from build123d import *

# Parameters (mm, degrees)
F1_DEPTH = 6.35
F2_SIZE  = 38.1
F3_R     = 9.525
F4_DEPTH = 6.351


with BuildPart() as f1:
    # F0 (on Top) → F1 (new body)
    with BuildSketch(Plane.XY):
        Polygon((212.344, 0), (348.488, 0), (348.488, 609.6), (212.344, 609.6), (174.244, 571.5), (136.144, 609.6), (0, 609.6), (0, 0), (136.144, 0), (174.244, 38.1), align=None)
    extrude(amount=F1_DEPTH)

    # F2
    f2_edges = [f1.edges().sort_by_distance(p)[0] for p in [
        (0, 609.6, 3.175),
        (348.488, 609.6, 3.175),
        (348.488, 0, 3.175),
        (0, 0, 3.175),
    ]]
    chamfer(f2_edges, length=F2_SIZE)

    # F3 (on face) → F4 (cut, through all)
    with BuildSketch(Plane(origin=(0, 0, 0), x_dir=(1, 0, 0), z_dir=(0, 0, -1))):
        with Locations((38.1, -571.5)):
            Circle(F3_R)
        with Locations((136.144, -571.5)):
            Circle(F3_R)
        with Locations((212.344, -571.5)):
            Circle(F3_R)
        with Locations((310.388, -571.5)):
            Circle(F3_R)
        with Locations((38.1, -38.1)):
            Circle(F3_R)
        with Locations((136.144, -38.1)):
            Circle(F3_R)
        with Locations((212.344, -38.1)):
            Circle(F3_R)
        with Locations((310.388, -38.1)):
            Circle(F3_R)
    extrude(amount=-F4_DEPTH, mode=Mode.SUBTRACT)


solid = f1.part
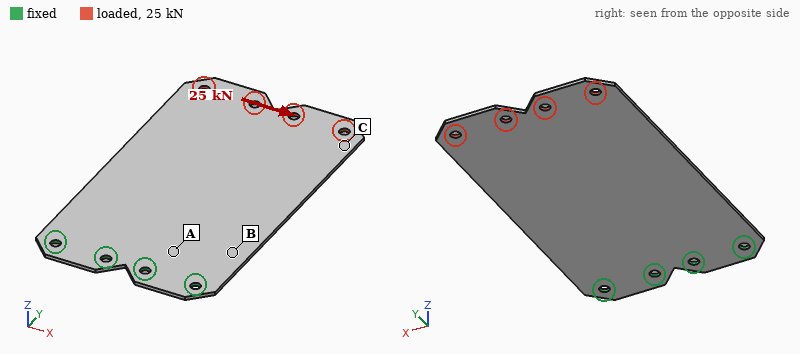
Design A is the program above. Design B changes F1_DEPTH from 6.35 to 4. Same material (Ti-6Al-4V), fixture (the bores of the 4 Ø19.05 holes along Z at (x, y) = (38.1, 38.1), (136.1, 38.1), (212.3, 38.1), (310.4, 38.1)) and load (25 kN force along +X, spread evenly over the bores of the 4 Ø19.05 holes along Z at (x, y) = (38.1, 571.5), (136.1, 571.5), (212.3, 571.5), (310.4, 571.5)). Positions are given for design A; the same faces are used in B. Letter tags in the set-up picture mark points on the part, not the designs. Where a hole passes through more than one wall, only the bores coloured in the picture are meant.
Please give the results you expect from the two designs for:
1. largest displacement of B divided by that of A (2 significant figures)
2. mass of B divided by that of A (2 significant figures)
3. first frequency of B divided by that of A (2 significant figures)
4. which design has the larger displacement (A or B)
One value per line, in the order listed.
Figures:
1.6
0.63
0.63
B
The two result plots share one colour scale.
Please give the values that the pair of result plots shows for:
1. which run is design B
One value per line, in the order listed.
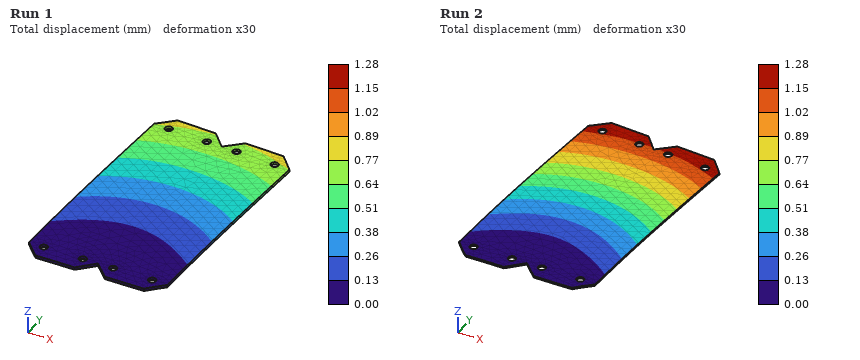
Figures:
Run 2
